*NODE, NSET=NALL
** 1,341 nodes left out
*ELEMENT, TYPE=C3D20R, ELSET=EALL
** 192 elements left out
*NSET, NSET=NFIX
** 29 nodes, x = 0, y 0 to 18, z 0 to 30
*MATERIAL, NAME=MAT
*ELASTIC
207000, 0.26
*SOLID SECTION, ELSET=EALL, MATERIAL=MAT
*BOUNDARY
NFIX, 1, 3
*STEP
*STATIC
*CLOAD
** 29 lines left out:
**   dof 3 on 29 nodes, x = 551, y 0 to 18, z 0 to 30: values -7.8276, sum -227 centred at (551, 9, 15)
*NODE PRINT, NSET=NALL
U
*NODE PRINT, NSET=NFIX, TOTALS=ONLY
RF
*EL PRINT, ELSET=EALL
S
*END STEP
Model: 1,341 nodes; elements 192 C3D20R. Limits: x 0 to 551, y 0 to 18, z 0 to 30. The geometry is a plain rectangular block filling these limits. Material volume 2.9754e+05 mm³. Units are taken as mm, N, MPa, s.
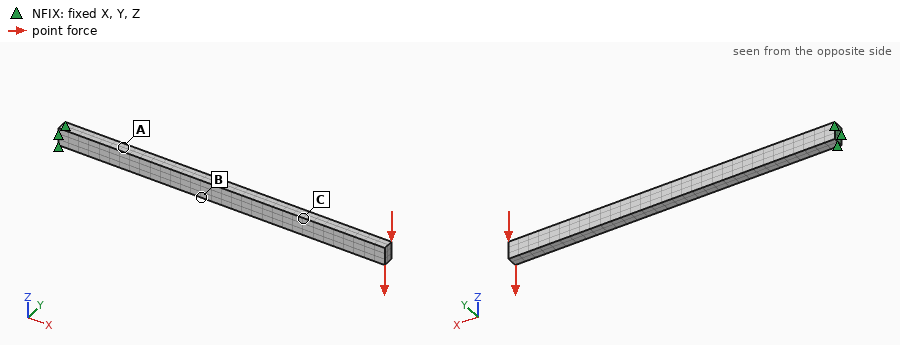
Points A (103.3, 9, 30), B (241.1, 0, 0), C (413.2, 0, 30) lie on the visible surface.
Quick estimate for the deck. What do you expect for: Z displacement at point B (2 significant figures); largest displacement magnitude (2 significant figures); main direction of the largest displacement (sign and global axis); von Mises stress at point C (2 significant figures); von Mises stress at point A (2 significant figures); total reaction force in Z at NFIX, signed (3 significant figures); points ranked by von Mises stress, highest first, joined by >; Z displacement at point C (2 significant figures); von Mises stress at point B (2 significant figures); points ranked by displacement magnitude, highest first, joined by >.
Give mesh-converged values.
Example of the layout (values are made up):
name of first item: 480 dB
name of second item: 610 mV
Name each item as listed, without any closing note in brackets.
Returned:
Z displacement at point B: -0.37 mm
largest displacement magnitude: 1.5 mm
main direction of the largest displacement: -Z
von Mises stress at point C: 12 MPa
von Mises stress at point A: 38 MPa
total reaction force in Z at NFIX, signed: 227 N
points ranked by von Mises stress, highest first, joined by >: A > B > C
Z displacement at point C: -0.96 mm
von Mises stress at point B: 26 MPa
points ranked by displacement magnitude, highest first, joined by >: C > B > A
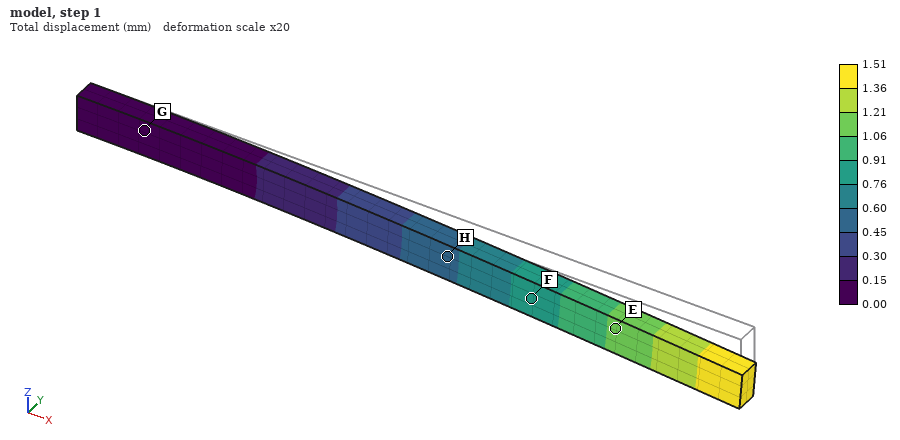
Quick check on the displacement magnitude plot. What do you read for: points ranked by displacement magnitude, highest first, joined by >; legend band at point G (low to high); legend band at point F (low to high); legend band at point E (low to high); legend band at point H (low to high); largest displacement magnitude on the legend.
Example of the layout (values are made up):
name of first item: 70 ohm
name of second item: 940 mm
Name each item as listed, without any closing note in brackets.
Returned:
points ranked by displacement magnitude, highest first, joined by >: E > F > H > G
legend band at point G: 0.00 to 0.15 mm
legend band at point F: 0.76 to 0.91 mm
legend band at point E: 1.06 to 1.21 mm
legend band at point H: 0.45 to 0.60 mm
largest displacement magnitude on the legend: 1.51 mm
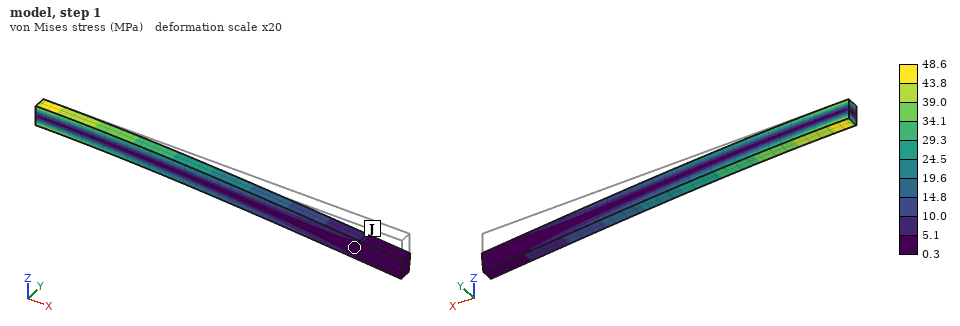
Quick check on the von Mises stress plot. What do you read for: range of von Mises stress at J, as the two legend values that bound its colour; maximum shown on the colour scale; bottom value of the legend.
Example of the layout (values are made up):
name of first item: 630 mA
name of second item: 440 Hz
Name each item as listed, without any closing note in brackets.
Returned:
range of von Mises stress at J, as the two legend values that bound its colour: 0.3 to 5.1 MPa
maximum shown on the colour scale: 48.6 MPa
bottom value of the legend: 0.3 MPa
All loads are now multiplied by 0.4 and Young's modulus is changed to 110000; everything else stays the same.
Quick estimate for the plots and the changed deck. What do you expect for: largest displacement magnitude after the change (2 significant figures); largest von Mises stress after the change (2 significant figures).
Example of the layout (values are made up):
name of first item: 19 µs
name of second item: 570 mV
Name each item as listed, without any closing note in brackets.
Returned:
largest displacement magnitude after the change: 1.1 mm
largest von Mises stress after the change: 19 MPa
